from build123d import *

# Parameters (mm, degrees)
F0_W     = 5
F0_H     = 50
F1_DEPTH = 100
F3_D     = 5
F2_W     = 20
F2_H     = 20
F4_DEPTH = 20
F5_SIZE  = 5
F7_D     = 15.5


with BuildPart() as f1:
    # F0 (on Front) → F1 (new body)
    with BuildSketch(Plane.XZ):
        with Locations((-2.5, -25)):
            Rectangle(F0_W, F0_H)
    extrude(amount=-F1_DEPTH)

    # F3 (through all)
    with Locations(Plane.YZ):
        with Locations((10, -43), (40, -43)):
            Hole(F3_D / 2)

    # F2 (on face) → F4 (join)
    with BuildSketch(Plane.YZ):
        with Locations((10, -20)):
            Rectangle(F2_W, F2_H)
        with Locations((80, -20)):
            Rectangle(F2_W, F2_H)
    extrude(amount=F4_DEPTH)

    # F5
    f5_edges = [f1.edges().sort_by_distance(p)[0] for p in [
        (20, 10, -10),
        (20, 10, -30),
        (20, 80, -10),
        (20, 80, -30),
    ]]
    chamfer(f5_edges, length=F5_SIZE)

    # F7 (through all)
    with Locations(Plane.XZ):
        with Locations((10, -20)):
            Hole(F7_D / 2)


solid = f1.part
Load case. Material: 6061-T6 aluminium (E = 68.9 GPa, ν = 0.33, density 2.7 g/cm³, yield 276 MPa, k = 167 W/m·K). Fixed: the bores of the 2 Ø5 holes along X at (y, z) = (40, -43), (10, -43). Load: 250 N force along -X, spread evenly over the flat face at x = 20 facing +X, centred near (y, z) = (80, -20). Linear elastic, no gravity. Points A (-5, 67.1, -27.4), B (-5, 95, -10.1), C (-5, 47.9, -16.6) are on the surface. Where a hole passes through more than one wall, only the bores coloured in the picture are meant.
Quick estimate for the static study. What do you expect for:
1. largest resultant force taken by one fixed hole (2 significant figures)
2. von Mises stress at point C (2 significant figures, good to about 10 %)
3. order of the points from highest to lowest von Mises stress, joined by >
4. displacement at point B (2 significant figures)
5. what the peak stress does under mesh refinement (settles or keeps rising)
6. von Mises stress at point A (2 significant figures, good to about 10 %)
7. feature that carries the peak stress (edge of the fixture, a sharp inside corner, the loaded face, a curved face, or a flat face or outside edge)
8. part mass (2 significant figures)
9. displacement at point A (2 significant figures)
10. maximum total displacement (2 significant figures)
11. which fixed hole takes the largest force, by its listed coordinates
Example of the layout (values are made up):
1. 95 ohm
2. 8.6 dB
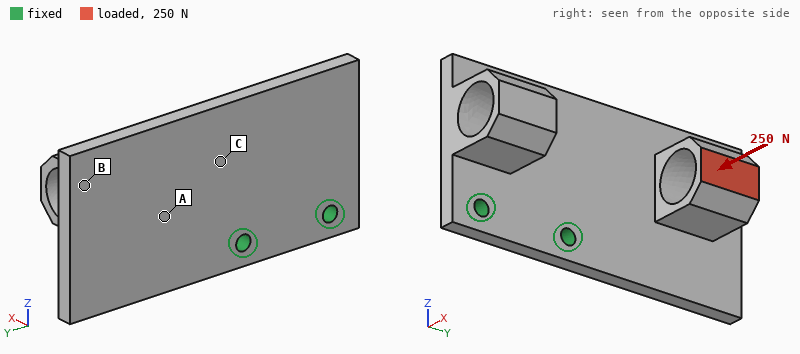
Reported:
1. 410 N
2. 30 MPa
3. C > A > B
4. 0.40 mm
5. keeps rising
6. 16 MPa
7. edge of the fixture
8. 87 g
9. 0.15 mm
10. 0.47 mm
11. (40, -43)
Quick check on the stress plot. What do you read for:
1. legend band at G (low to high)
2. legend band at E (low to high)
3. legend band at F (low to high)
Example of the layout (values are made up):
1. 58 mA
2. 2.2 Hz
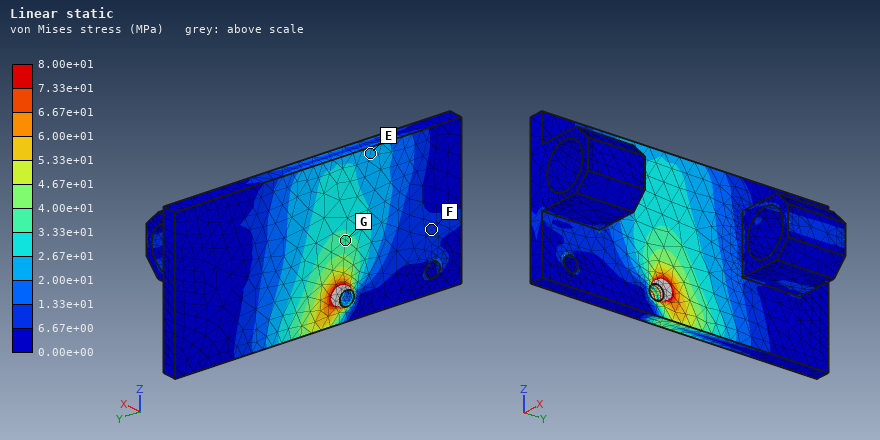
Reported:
1. 3.33e+01 to 4.00e+01 MPa
2. 2.00e+01 to 2.67e+01 MPa
3. 6.67e+00 to 1.33e+01 MPa
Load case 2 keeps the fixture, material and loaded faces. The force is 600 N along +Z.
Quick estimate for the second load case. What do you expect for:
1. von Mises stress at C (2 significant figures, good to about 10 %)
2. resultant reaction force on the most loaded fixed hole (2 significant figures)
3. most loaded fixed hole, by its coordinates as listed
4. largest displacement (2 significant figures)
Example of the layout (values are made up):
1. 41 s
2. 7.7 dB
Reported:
1. 34 MPa
2. 1.3 kN
3. (40, -43)
4. 0.44 mm
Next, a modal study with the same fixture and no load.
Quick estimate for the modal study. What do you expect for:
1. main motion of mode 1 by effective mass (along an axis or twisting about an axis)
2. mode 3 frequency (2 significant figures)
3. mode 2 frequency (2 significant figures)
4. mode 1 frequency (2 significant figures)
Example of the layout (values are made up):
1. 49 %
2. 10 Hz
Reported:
1. along X
2. 2700 Hz
3. 1600 Hz
4. 770 Hz
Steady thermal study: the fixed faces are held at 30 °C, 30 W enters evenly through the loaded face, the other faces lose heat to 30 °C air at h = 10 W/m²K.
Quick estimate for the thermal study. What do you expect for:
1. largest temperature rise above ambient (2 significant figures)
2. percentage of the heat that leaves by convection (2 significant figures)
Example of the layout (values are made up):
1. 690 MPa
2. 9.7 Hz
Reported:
1. 66 K
2. 10 %
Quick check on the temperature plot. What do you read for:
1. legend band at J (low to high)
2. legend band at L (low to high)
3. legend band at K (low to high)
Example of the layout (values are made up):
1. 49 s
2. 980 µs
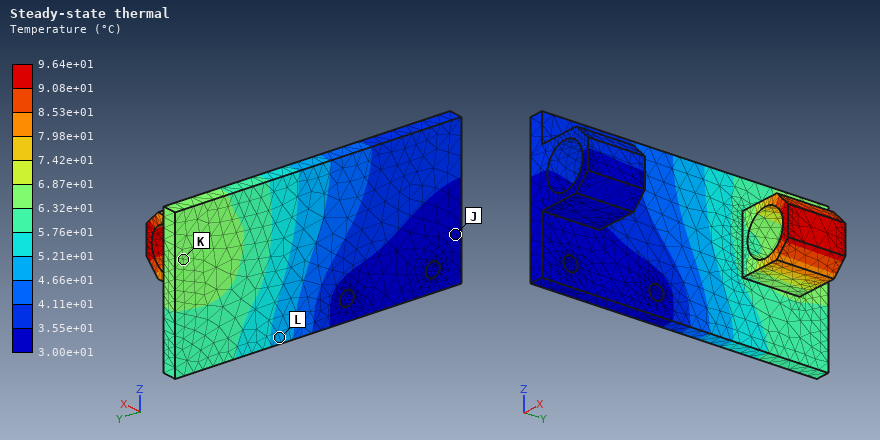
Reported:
1. 3.00e+01 to 3.55e+01 °C
2. 4.66e+01 to 5.21e+01 °C
3. 6.32e+01 to 6.87e+01 °C
